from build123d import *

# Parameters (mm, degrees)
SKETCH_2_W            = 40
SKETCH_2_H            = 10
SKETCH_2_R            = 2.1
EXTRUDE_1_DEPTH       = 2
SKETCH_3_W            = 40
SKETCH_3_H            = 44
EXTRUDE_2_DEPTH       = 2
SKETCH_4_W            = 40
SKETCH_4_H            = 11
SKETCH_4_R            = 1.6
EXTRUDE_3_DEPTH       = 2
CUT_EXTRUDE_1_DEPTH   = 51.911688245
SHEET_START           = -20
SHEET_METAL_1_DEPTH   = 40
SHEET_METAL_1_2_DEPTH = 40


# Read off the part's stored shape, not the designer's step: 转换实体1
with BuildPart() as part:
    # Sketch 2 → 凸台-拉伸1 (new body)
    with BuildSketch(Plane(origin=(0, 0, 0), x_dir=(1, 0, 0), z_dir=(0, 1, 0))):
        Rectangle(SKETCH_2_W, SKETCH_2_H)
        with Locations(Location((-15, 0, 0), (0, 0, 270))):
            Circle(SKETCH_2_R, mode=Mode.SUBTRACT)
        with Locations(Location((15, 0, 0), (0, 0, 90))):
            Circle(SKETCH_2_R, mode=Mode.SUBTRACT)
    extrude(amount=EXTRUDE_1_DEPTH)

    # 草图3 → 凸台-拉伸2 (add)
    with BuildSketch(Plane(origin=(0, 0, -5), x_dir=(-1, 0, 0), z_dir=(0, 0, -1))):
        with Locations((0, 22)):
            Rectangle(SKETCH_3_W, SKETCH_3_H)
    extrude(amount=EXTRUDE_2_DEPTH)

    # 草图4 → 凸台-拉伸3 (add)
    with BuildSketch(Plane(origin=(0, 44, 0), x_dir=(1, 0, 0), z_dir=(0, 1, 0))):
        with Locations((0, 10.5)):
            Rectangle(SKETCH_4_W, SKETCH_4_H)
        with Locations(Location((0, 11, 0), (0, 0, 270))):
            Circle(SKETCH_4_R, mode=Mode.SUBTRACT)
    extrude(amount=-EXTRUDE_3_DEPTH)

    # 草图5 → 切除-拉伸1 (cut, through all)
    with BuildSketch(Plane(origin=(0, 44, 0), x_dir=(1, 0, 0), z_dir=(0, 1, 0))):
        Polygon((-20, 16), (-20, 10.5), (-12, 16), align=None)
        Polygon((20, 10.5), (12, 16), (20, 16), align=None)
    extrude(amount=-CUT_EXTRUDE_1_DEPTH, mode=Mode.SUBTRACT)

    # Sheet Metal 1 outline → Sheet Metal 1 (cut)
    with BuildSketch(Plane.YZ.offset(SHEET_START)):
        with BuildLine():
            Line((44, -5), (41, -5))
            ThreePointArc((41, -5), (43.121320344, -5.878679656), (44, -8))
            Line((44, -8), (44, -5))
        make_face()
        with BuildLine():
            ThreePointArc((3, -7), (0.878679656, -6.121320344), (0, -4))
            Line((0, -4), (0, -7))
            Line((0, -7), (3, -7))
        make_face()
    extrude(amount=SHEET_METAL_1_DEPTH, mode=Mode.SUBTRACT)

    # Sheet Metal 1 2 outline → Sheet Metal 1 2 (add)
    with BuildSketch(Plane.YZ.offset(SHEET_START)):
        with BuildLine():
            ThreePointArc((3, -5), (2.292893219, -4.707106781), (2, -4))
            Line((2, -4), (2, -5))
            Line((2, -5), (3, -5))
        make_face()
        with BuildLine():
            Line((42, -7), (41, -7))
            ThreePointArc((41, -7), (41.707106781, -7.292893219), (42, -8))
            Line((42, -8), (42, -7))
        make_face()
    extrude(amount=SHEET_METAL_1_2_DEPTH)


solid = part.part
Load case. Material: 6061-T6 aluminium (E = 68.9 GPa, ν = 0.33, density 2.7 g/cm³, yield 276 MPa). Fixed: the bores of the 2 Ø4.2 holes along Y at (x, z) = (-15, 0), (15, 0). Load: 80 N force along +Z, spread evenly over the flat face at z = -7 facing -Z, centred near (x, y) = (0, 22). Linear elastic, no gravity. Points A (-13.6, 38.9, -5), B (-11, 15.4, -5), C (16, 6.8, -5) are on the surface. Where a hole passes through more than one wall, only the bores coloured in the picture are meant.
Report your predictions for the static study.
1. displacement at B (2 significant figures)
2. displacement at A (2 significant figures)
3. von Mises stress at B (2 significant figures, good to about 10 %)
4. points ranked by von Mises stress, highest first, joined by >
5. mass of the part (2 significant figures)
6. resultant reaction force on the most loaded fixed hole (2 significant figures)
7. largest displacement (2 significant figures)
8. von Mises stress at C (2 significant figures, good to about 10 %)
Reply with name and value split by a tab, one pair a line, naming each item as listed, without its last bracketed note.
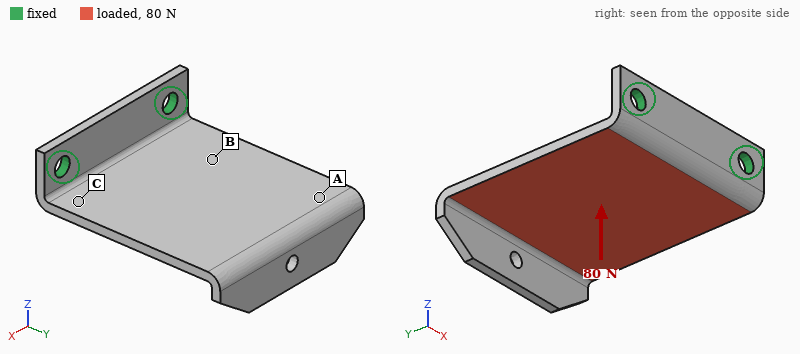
displacement at B	0.14 mm
displacement at A	0.49 mm
von Mises stress at B	24 MPa
points ranked by von Mises stress, highest first, joined by >	C > B > A
mass of the part	13 g
resultant reaction force on the most loaded fixed hole	41 N
largest displacement	0.60 mm
von Mises stress at C	42 MPa
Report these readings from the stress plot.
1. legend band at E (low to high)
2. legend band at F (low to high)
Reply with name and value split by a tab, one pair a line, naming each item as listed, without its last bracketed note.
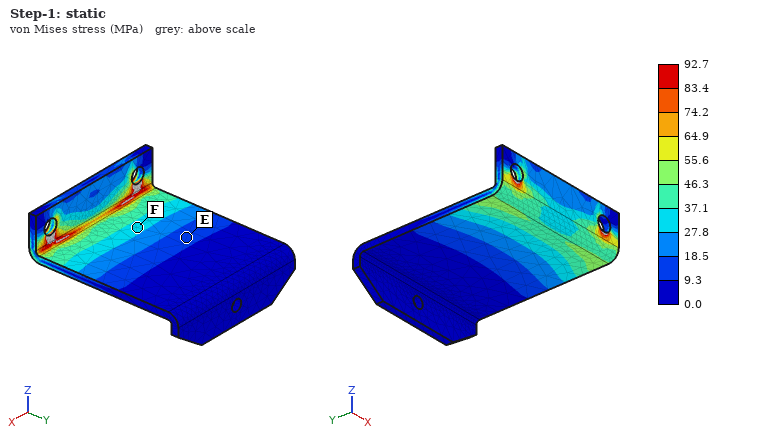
legend band at E	9.3 to 18.5 MPa
legend band at F	27.8 to 37.1 MPa
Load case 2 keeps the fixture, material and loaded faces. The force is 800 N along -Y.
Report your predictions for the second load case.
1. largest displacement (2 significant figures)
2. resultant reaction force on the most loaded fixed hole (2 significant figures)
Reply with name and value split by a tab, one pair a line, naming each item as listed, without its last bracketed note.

largest displacement	0.67 mm
resultant reaction force on the most loaded fixed hole	400 N
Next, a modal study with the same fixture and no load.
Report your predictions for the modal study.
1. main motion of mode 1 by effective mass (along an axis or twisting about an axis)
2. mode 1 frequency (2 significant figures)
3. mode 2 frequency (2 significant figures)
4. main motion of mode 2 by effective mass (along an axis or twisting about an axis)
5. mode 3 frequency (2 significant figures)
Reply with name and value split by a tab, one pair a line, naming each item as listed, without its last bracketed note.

main motion of mode 1 by effective mass	along Z
mode 1 frequency	590 Hz
mode 2 frequency	1800 Hz
main motion of mode 2 by effective mass	twisting about Y
mode 3 frequency	3900 Hz
